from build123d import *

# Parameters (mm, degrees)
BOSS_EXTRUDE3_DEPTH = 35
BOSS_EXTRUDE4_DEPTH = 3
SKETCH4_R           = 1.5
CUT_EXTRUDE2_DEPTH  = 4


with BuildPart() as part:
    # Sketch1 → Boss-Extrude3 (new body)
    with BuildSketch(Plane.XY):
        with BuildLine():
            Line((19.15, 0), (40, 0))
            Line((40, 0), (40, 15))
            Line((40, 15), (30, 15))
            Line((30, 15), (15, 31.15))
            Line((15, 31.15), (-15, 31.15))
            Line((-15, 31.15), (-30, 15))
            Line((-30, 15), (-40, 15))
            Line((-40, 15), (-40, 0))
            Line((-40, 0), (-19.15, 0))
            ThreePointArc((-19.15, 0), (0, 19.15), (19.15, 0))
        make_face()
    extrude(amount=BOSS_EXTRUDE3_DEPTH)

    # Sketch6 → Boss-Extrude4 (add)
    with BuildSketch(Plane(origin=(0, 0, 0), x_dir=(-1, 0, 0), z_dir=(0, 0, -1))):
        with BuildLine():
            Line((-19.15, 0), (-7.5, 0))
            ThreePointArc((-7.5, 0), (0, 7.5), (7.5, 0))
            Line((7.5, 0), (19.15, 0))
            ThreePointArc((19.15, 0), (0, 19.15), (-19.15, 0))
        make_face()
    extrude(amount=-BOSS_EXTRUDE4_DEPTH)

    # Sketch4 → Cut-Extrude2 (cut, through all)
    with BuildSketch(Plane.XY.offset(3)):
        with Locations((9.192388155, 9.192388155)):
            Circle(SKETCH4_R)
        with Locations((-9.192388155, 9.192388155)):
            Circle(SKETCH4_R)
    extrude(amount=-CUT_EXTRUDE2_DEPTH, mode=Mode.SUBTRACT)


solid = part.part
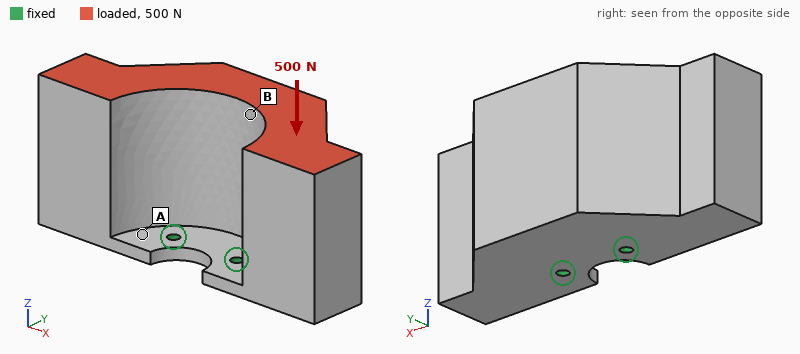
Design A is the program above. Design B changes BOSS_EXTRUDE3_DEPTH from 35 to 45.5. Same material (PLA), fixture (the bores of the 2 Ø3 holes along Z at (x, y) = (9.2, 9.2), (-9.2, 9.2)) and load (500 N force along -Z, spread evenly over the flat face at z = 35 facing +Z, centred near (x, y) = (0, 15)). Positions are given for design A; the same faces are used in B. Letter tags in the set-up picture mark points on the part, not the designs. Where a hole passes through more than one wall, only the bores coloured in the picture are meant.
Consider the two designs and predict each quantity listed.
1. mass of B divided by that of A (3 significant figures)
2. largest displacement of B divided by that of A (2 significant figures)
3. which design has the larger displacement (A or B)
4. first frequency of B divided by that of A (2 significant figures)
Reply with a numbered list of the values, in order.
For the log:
1. 1.29
2. 1.2
3. B
4. 0.70
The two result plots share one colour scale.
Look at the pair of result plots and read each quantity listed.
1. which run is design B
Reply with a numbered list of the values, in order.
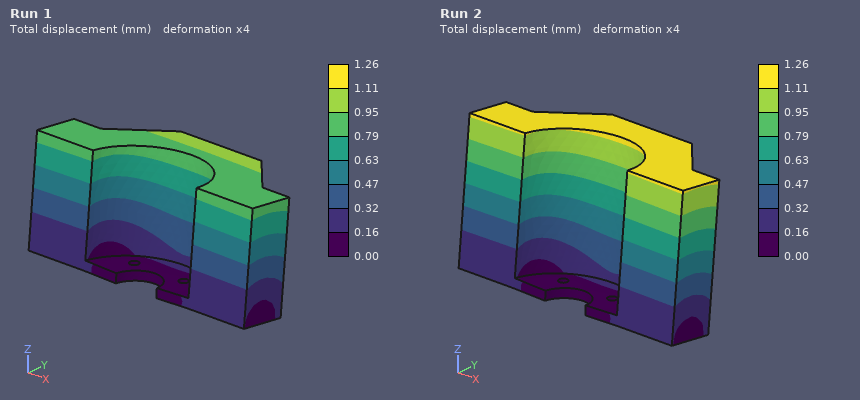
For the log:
1. Run 2
